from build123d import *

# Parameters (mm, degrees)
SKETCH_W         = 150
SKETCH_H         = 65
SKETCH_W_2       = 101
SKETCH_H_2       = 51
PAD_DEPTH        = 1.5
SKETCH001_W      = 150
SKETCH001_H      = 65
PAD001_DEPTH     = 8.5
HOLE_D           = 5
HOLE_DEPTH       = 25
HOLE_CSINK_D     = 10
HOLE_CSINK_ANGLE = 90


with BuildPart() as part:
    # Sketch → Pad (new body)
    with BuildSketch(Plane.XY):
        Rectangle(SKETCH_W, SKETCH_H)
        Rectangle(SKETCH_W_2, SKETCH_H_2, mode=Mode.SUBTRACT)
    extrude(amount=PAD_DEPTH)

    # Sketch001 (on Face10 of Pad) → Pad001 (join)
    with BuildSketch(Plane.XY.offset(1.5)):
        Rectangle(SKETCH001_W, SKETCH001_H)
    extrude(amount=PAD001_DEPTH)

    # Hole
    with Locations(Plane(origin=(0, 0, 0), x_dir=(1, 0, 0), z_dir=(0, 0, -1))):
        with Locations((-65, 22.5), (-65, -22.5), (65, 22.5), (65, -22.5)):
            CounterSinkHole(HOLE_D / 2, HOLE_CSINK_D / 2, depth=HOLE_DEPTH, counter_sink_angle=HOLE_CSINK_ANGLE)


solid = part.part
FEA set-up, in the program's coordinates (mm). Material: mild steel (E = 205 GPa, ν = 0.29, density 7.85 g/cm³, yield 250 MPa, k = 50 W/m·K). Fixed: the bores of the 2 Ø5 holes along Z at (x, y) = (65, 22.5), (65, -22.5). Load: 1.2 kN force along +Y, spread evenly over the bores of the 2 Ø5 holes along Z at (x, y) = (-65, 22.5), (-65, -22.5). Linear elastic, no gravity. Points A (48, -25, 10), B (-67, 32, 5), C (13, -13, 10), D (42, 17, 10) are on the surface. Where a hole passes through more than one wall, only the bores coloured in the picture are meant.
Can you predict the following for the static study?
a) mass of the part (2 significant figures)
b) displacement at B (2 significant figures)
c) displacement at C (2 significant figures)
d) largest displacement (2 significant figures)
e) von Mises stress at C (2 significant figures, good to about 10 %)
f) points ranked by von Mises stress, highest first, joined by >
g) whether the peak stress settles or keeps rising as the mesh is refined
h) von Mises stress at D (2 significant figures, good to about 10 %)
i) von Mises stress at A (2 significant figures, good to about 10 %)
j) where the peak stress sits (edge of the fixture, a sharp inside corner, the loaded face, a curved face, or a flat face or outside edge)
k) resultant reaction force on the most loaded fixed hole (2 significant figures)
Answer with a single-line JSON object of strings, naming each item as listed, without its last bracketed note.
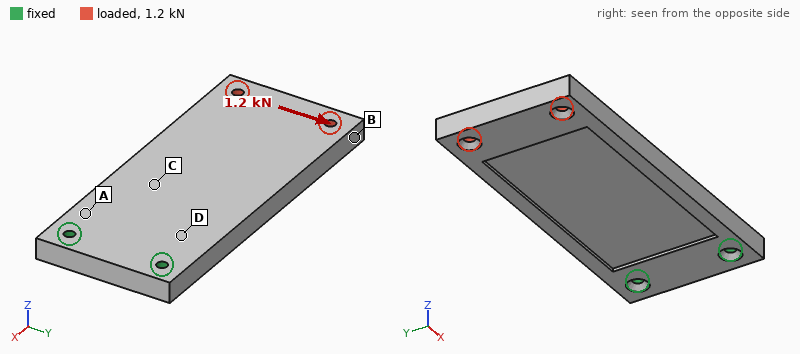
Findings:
{"mass of the part": "700 g", "displacement at B": "29 µm", "displacement at C": "7.2 µm", "largest displacement": "31 µm", "von Mises stress at C": "7.8 MPa", "points ranked by von Mises stress, highest first, joined by >": "A > D > C > B", "whether the peak stress settles or keeps rising as the mesh is refined": "keeps rising", "von Mises stress at D": "12 MPa", "von Mises stress at A": "17 MPa", "where the peak stress sits": "edge of the fixture", "resultant reaction force on the most loaded fixed hole": "3.4 kN"}
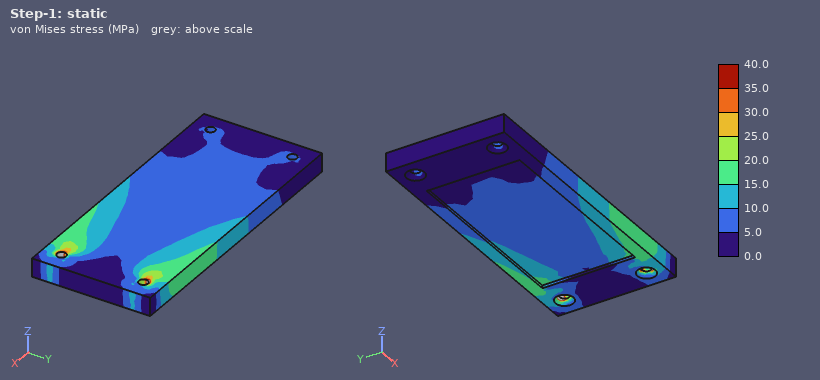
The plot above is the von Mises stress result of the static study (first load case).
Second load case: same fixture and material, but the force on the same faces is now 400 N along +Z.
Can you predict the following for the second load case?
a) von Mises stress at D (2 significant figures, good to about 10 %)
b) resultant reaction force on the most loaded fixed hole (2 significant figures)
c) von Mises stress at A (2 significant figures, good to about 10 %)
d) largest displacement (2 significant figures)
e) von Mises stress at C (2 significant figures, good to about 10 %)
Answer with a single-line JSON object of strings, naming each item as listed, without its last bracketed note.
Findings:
{"von Mises stress at D": "46 MPa", "resultant reaction force on the most loaded fixed hole": "280 N", "von Mises stress at A": "52 MPa", "largest displacement": "0.44 mm", "von Mises stress at C": "35 MPa"}
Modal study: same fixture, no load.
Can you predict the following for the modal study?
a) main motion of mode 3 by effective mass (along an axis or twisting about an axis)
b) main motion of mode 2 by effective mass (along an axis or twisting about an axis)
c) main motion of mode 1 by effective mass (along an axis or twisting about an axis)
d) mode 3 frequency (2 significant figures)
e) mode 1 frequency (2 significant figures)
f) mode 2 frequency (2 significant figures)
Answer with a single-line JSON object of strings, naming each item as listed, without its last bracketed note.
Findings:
{"main motion of mode 3 by effective mass": "along Z", "main motion of mode 2 by effective mass": "twisting about X", "main motion of mode 1 by effective mass": "along Z", "mode 3 frequency": "2200 Hz", "mode 1 frequency": "360 Hz", "mode 2 frequency": "1600 Hz"}
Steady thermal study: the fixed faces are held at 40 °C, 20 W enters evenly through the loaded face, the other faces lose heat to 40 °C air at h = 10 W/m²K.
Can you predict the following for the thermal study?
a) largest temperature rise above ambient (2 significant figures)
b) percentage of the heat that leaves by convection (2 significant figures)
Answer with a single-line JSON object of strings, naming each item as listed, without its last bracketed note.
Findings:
{"largest temperature rise above ambient": "72 K", "percentage of the heat that leaves by convection": "39 %"}
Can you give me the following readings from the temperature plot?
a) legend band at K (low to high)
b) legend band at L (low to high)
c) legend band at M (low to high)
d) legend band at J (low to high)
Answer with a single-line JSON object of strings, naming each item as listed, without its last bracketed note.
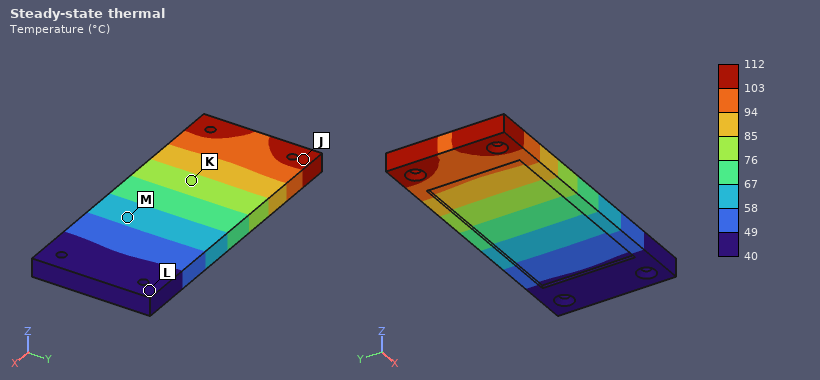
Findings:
{"legend band at K": "76 to 85 °C", "legend band at L": "40 to 49 °C", "legend band at M": "58 to 67 °C", "legend band at J": "103 to 112 °C"}
